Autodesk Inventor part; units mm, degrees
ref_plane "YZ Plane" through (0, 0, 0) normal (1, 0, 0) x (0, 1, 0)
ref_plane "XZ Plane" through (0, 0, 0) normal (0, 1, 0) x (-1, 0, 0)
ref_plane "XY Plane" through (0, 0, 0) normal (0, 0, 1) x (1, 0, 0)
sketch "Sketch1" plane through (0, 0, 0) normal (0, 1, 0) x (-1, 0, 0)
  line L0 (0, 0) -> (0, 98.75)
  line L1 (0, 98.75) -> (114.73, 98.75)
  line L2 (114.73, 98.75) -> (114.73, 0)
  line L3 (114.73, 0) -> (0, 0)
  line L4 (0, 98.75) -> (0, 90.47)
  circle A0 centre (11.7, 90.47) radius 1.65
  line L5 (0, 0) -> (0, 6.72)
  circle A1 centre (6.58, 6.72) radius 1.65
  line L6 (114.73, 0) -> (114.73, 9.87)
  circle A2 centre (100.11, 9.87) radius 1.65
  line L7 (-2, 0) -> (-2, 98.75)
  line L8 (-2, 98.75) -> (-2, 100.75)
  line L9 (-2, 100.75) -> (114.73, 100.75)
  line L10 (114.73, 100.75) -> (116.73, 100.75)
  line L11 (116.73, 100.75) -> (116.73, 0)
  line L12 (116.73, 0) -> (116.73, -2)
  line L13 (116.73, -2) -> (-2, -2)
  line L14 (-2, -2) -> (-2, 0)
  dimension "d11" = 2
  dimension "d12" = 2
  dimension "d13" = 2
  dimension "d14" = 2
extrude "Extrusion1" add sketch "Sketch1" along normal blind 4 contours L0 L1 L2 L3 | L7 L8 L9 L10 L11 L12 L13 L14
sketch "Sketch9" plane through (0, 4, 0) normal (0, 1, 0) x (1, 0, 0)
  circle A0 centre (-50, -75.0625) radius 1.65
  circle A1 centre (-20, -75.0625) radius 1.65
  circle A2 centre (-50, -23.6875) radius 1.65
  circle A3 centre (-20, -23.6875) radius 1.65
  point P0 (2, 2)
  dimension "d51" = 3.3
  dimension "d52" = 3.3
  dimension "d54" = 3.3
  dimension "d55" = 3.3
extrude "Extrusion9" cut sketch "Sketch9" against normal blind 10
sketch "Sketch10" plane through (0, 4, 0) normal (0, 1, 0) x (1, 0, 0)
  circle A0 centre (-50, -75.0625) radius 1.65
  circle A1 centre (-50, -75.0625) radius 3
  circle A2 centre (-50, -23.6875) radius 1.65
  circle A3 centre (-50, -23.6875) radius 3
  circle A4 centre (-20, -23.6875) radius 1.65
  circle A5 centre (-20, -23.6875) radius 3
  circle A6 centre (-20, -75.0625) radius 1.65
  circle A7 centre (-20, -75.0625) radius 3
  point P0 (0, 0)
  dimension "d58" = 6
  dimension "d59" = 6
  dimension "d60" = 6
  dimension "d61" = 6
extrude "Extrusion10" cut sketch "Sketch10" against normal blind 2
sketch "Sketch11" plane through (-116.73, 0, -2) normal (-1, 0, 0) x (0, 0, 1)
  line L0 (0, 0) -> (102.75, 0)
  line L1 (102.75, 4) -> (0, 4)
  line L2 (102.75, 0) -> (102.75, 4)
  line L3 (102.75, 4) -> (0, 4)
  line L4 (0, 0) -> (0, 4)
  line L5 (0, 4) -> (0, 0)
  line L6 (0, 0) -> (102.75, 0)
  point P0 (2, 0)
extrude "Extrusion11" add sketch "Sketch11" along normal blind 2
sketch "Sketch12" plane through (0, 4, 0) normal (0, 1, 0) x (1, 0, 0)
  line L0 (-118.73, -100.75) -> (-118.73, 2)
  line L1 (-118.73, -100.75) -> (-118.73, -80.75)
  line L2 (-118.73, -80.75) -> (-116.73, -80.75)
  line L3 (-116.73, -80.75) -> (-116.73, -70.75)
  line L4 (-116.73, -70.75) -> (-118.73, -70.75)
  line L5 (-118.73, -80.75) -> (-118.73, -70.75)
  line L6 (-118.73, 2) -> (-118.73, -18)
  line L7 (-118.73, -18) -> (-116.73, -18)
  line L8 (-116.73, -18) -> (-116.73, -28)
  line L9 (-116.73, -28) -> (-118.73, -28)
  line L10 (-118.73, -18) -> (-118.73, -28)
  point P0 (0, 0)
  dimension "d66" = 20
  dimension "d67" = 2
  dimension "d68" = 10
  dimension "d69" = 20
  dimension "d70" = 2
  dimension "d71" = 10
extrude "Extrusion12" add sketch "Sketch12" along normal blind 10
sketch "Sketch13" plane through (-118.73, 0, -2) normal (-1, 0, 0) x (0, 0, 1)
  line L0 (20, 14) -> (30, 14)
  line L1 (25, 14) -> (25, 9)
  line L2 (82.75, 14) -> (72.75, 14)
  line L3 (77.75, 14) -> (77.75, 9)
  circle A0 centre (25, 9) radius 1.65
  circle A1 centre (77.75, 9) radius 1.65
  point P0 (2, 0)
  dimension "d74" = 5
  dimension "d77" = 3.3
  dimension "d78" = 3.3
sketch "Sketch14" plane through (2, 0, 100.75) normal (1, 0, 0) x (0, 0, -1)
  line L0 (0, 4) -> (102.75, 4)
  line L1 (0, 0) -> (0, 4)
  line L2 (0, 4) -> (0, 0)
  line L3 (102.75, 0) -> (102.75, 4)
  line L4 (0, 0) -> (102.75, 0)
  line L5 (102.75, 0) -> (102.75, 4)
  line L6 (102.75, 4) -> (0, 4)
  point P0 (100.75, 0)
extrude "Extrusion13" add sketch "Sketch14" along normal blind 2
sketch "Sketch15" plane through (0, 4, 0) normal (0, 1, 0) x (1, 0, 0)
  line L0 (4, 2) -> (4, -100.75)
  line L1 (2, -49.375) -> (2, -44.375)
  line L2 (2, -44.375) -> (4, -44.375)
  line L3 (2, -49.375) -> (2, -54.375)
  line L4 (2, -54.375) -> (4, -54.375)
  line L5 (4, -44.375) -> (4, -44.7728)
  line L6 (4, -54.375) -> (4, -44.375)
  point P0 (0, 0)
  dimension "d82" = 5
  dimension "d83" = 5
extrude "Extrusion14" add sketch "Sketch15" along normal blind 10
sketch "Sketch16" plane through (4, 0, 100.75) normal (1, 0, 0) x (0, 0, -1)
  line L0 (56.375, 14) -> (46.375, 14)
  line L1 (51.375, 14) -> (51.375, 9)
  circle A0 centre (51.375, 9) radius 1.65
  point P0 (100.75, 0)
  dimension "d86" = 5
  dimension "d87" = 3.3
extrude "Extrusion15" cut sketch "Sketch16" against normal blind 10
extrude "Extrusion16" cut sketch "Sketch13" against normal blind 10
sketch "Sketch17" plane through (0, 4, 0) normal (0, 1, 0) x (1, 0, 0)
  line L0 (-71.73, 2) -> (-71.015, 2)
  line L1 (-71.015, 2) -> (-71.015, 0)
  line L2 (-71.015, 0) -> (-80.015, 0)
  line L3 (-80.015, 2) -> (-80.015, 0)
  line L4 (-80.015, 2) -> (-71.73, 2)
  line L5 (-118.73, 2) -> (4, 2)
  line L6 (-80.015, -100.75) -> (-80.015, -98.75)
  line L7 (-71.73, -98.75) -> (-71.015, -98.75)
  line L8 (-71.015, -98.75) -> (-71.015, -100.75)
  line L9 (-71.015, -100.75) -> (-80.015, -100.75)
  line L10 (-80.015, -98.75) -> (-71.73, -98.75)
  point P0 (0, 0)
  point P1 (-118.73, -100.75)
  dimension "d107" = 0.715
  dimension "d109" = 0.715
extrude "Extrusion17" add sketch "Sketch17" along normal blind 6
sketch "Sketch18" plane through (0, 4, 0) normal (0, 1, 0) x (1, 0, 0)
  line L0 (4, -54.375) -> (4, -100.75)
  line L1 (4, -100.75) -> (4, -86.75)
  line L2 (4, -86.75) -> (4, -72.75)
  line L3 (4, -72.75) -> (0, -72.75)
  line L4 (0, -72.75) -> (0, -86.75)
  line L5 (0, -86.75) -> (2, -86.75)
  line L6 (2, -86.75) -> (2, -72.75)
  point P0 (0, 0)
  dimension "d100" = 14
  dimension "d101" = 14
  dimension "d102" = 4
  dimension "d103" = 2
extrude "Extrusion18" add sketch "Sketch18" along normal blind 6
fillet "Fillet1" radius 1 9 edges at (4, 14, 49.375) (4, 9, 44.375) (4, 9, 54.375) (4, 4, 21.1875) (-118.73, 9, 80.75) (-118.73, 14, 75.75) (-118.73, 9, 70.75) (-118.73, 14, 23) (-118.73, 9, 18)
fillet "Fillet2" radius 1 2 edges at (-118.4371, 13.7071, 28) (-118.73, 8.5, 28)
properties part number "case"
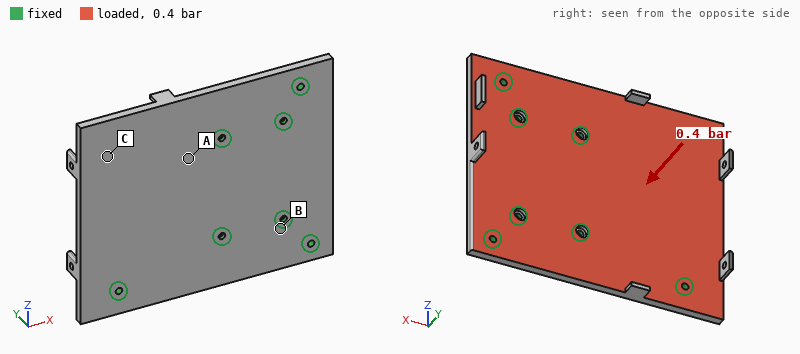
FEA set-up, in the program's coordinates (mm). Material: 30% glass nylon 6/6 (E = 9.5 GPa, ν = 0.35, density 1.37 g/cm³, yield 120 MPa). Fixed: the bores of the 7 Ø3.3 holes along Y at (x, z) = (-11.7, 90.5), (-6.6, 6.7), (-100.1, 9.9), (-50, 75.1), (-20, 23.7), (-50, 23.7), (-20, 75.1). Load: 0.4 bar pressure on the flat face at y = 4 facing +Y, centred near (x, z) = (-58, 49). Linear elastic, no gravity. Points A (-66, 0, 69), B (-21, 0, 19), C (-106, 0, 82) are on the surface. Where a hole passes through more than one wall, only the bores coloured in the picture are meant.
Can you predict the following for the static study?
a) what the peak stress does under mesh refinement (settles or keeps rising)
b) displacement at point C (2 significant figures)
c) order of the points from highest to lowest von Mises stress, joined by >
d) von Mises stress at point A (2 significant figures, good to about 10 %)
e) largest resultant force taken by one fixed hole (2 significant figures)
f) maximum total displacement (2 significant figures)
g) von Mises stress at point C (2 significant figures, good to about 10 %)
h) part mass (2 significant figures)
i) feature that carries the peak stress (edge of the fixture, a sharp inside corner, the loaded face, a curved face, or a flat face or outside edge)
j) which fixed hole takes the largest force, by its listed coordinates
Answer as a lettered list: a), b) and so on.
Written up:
a) keeps rising
b) 1.0 mm
c) A > C > B
d) 10 MPa
e) 280 N
f) 1.6 mm
g) 5.1 MPa
h) 70 g
i) edge of the fixture
j) (-50, 75.1)
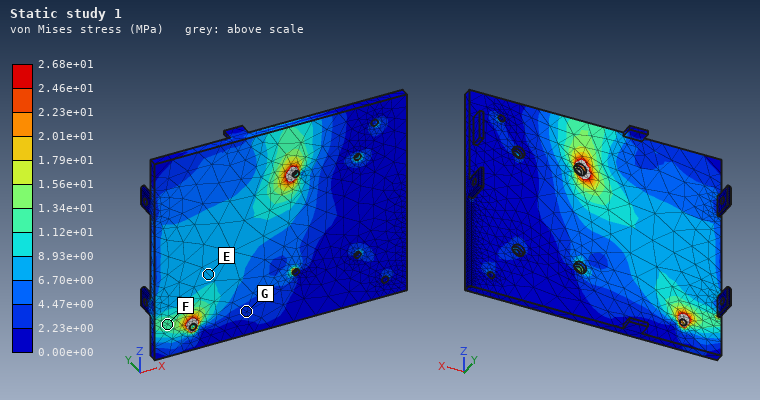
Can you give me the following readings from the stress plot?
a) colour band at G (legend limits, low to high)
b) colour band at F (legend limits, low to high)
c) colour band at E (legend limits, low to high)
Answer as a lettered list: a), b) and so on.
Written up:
a) 2.23e+00 to 4.47e+00 MPa
b) 1.12e+01 to 1.34e+01 MPa
c) 6.70e+00 to 8.93e+00 MPa
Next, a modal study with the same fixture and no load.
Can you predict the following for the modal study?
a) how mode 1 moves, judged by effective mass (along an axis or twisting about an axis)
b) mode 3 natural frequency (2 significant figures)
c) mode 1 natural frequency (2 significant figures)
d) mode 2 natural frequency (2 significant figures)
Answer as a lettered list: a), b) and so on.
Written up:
a) along Y
b) 1900 Hz
c) 480 Hz
d) 1300 Hz
